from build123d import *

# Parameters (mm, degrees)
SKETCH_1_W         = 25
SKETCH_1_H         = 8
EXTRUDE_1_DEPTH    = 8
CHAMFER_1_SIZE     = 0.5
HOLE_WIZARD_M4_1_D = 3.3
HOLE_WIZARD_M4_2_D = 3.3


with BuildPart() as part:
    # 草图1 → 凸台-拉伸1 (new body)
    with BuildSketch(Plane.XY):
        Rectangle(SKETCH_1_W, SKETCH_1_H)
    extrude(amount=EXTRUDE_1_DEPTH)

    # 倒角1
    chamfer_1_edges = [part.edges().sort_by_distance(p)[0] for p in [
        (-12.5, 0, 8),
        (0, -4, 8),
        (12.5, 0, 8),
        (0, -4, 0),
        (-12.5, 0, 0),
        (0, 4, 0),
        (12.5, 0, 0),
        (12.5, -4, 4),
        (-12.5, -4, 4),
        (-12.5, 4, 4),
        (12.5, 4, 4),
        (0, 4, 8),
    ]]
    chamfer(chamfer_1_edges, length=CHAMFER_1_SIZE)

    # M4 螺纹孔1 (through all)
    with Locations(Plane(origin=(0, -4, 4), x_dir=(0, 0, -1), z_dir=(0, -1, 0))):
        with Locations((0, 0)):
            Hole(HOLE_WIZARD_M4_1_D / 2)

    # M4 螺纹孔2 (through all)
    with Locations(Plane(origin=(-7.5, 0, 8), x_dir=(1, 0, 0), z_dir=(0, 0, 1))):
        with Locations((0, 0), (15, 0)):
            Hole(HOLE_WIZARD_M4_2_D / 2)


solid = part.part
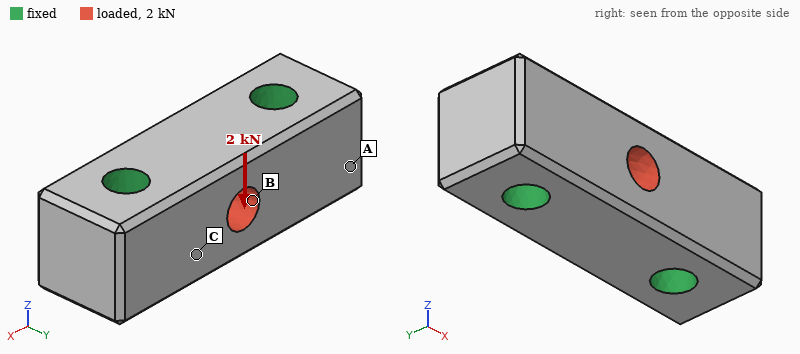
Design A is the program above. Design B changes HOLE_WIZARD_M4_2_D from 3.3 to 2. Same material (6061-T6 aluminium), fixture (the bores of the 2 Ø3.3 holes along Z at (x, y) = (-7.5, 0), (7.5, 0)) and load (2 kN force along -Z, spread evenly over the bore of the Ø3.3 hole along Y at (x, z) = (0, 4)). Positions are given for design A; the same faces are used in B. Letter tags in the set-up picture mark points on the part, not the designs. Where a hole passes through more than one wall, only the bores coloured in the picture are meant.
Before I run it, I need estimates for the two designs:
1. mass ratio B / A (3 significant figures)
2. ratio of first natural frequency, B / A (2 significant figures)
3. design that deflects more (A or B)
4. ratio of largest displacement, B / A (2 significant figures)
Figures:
1.06
0.73
B
1.2
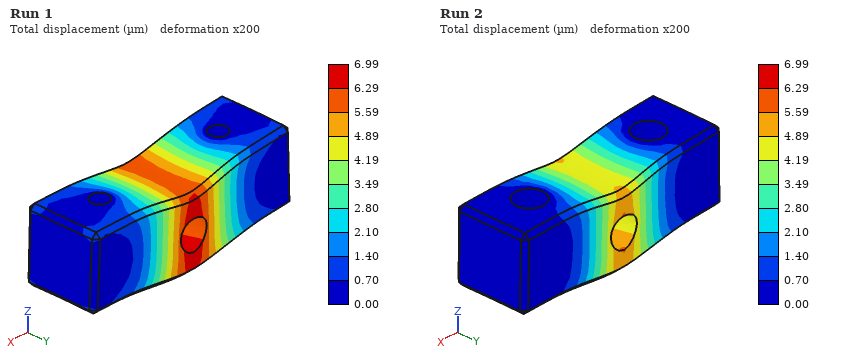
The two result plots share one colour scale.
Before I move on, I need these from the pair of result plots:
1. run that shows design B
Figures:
Run 1
